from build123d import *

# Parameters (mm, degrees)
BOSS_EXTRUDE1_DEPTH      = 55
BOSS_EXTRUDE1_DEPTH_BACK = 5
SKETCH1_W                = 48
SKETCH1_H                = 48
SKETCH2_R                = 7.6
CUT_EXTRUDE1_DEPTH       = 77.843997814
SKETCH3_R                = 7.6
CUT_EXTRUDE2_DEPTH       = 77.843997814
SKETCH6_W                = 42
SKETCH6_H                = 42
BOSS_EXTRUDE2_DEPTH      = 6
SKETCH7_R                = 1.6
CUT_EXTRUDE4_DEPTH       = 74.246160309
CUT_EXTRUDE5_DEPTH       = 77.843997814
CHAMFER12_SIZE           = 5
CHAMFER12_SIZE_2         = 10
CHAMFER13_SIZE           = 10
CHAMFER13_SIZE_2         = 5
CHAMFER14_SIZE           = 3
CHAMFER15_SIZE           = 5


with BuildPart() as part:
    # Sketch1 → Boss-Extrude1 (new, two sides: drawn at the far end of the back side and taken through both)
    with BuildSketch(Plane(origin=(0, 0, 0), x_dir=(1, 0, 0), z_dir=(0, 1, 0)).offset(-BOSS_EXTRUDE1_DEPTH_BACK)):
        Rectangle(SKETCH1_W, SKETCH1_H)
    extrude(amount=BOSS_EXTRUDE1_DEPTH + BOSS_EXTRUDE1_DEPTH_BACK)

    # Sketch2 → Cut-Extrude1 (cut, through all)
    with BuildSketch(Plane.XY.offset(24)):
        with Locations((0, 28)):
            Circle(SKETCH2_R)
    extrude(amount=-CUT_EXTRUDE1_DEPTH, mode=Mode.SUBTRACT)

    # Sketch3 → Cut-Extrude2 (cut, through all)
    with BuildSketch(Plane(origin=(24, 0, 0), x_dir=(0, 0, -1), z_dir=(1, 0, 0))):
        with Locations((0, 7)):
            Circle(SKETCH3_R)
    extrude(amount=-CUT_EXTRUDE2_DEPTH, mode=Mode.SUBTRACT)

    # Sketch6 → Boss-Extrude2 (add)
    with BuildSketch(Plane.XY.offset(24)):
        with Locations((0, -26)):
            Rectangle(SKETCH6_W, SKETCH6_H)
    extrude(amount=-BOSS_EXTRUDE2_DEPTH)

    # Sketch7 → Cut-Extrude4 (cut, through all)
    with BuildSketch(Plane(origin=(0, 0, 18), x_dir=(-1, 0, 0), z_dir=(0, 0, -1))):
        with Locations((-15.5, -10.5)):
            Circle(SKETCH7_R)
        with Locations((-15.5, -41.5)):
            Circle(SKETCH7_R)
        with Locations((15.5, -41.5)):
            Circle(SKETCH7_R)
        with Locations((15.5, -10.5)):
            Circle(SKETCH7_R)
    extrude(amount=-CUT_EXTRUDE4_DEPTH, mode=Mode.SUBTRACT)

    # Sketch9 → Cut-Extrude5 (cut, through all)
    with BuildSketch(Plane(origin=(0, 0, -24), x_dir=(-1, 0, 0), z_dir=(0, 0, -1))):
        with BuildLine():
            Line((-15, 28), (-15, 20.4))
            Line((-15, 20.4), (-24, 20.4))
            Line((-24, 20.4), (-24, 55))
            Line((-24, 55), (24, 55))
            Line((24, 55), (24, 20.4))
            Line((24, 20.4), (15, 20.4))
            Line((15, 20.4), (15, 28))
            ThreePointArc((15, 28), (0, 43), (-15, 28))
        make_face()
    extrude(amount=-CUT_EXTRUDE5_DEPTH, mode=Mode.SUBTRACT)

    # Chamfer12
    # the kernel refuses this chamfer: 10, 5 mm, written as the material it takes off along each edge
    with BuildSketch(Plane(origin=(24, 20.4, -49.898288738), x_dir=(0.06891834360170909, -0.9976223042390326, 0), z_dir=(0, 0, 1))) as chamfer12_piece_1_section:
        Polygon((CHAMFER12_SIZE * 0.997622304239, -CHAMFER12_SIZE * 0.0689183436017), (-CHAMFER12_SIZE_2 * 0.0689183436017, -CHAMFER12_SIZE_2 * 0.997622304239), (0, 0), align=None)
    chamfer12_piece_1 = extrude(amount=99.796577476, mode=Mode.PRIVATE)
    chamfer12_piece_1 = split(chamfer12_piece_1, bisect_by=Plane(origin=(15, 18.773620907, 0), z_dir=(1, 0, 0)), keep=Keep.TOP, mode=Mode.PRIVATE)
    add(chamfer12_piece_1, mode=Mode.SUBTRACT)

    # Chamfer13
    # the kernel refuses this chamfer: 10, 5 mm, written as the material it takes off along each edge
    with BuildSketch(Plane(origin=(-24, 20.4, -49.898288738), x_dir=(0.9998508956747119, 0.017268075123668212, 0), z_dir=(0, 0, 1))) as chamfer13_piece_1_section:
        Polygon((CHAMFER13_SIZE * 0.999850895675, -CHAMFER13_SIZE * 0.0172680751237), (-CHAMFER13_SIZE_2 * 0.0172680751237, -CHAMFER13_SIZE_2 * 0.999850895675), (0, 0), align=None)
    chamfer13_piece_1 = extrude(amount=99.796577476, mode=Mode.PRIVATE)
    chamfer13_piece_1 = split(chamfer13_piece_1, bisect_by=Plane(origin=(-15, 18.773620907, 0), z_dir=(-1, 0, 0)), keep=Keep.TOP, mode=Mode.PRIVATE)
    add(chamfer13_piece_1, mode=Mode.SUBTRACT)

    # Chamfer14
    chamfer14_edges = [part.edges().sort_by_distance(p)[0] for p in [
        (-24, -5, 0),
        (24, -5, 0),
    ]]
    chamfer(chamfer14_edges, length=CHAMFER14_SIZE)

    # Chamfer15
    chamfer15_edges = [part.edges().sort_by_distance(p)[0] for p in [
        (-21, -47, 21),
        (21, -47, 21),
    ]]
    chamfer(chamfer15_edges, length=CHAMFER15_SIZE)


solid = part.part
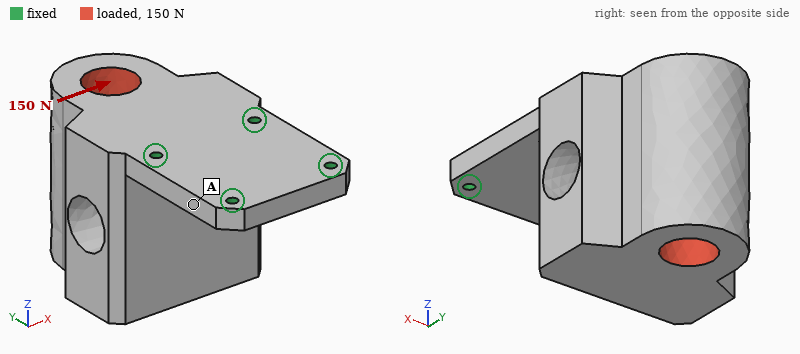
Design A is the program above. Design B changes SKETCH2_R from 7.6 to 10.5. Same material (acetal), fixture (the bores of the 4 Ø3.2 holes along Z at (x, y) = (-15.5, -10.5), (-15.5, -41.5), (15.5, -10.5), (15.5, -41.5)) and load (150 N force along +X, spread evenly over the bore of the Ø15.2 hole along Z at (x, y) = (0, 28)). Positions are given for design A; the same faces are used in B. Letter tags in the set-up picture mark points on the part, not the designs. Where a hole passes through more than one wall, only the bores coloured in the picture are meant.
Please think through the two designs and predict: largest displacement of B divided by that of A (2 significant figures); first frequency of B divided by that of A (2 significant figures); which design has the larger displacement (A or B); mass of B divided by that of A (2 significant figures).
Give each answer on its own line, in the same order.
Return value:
1.1
1.1
B
0.90
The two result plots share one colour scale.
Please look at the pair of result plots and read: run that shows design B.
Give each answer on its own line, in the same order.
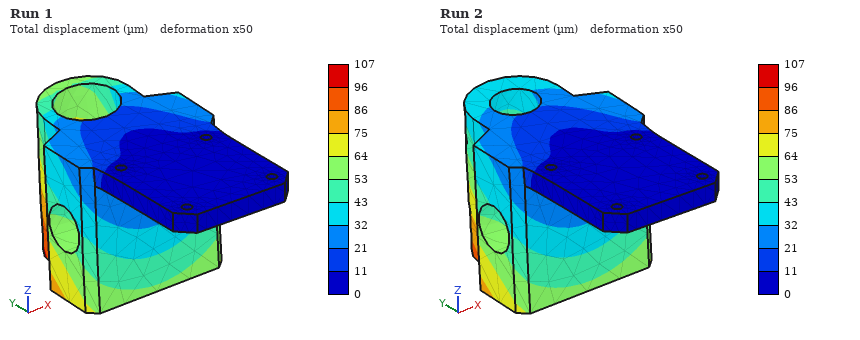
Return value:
Run 1
